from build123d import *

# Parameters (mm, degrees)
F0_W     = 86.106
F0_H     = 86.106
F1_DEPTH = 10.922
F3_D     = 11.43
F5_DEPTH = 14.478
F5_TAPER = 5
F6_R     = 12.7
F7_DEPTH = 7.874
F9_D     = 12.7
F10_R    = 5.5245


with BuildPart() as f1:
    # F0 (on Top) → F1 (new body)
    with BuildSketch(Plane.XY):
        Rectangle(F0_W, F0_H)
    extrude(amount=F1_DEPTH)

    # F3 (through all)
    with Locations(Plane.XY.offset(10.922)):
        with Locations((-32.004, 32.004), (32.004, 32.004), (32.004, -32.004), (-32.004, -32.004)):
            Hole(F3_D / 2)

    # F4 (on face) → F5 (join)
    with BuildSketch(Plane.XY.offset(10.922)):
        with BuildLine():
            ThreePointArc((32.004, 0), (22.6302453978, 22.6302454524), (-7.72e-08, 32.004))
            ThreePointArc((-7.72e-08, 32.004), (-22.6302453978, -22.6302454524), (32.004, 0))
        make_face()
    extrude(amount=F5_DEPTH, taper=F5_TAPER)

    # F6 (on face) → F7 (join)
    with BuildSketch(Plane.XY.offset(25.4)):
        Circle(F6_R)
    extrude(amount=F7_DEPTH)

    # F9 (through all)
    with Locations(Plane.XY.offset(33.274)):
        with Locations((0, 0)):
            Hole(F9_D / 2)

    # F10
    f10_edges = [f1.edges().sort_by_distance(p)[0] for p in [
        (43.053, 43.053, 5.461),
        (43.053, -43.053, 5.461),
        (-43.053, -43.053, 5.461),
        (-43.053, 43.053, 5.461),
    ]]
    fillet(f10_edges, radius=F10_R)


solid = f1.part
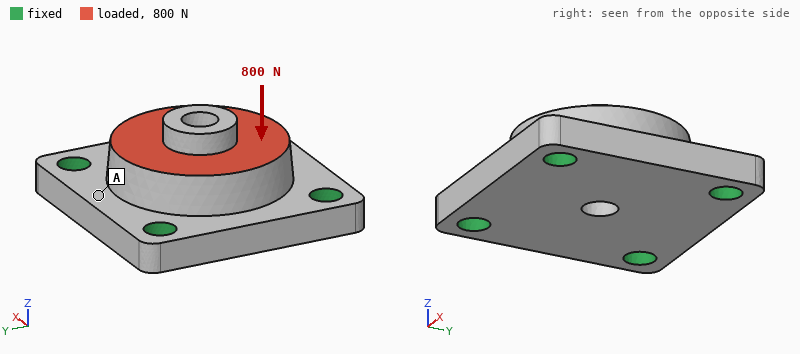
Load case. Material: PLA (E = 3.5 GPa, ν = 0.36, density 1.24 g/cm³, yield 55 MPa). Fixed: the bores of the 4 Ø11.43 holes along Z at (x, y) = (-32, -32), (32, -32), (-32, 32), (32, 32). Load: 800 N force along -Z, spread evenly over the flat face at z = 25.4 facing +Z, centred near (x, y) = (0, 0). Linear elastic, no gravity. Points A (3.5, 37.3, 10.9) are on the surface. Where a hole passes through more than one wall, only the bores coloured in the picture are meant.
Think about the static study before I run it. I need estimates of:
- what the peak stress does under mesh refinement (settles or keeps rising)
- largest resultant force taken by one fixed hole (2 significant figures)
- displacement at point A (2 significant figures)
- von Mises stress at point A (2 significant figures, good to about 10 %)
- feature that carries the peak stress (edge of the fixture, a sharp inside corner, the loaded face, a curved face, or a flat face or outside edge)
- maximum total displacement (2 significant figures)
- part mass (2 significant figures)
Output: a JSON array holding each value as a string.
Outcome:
["keeps rising", "220 N", "12 µm", "0.63 MPa", "edge of the fixture", "17 µm", "150 g"]
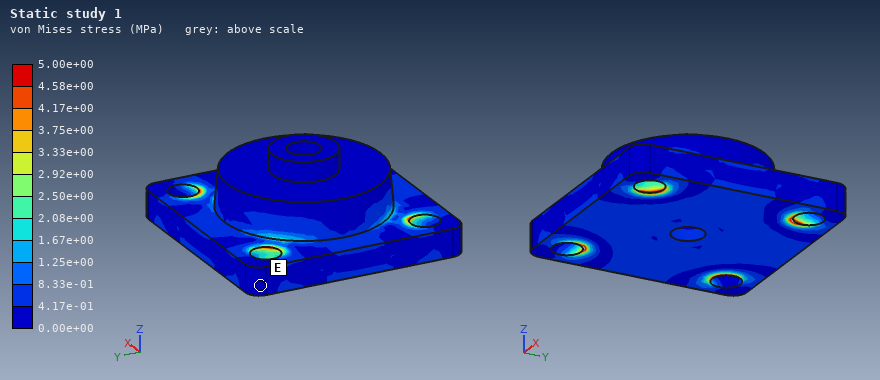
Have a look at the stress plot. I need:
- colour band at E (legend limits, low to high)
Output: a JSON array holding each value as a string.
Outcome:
["0.00e+00 to 4.17e-01 MPa"]
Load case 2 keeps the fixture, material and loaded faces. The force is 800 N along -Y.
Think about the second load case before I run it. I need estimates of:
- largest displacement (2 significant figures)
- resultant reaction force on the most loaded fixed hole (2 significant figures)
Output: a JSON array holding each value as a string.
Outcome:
["21 µm", "260 N"]
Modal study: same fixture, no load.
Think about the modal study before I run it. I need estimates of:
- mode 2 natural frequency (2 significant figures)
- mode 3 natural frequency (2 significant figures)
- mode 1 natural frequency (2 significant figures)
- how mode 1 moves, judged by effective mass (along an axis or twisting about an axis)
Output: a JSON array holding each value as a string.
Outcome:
["4400 Hz", "4400 Hz", "3400 Hz", "along Z"]
